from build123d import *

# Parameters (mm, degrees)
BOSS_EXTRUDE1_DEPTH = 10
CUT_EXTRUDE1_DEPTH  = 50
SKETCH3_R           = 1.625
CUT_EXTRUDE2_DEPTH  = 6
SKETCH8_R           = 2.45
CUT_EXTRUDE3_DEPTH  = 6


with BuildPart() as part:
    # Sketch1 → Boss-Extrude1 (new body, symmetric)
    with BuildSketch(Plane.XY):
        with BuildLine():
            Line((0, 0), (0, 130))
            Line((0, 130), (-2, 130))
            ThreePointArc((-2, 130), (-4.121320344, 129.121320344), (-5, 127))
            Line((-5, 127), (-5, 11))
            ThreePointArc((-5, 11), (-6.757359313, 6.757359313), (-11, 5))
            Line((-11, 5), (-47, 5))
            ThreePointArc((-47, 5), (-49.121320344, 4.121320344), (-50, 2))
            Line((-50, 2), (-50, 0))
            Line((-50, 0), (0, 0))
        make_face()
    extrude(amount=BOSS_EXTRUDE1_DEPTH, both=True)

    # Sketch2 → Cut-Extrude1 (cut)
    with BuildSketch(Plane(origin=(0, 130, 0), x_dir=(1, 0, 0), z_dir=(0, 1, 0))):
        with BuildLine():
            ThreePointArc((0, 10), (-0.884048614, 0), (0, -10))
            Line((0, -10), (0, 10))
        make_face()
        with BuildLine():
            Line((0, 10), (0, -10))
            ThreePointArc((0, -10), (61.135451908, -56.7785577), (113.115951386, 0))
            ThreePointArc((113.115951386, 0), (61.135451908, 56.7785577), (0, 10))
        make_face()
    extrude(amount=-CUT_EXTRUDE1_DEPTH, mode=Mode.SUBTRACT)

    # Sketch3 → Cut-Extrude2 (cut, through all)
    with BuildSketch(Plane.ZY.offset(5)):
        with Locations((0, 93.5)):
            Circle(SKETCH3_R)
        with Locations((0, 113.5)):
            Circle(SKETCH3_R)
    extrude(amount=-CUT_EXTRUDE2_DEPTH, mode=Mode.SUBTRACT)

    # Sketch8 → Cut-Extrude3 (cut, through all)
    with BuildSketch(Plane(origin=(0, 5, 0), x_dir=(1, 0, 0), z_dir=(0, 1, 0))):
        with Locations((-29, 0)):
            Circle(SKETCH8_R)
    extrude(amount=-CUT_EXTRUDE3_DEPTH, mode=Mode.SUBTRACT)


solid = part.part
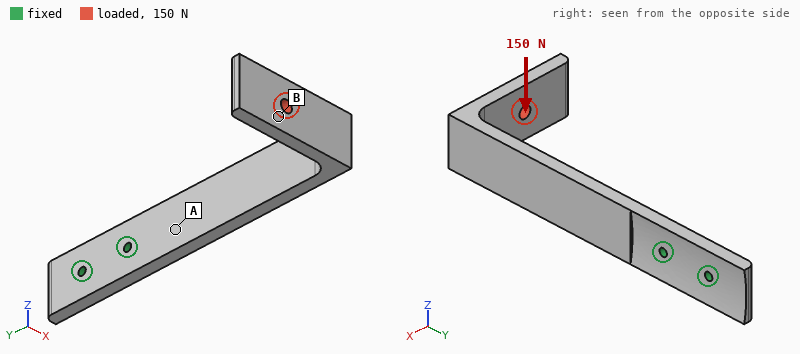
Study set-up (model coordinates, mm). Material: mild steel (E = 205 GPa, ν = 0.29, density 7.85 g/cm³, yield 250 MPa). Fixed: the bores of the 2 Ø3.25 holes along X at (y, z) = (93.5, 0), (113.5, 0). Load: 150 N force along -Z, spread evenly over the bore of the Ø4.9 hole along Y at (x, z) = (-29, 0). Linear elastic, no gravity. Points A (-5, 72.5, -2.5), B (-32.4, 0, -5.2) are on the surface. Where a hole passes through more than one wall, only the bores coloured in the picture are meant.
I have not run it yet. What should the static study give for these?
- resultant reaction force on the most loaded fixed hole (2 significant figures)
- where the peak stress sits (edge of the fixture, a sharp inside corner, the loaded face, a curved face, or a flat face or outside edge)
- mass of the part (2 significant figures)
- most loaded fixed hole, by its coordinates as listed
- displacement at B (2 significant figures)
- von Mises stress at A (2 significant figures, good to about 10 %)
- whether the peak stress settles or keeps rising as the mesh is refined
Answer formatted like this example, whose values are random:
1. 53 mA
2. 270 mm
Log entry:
1. 700 N
2. edge of the fixture
3. 130 g
4. (93.5, 0)
5. 0.28 mm
6. 55 MPa
7. keeps rising
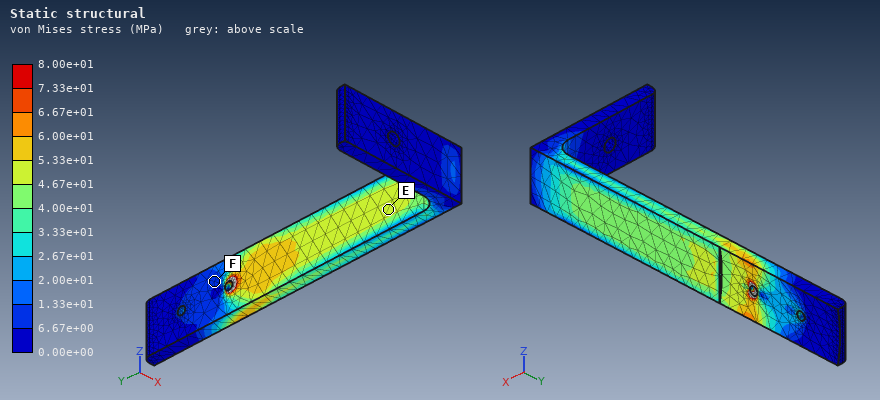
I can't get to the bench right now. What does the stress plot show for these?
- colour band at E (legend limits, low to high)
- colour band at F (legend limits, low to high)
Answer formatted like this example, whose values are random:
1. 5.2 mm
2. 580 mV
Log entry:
1. 4.67e+01 to 5.33e+01 MPa
2. 6.67e+00 to 1.33e+01 MPa
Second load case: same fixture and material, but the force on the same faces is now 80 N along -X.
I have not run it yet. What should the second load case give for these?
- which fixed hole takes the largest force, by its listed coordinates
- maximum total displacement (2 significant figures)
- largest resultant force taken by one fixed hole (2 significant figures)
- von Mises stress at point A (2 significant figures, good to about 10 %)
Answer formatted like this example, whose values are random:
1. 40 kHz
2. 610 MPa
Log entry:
1. (93.5, 0)
2. 0.73 mm
3. 230 N
4. 68 MPa
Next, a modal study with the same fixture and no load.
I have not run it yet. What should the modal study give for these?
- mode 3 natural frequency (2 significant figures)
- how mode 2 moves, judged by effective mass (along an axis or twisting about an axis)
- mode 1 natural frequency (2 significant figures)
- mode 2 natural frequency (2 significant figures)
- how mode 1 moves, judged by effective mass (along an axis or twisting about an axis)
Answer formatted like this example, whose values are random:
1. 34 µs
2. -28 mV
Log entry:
1. 1100 Hz
2. along Z
3. 240 Hz
4. 620 Hz
5. along X
